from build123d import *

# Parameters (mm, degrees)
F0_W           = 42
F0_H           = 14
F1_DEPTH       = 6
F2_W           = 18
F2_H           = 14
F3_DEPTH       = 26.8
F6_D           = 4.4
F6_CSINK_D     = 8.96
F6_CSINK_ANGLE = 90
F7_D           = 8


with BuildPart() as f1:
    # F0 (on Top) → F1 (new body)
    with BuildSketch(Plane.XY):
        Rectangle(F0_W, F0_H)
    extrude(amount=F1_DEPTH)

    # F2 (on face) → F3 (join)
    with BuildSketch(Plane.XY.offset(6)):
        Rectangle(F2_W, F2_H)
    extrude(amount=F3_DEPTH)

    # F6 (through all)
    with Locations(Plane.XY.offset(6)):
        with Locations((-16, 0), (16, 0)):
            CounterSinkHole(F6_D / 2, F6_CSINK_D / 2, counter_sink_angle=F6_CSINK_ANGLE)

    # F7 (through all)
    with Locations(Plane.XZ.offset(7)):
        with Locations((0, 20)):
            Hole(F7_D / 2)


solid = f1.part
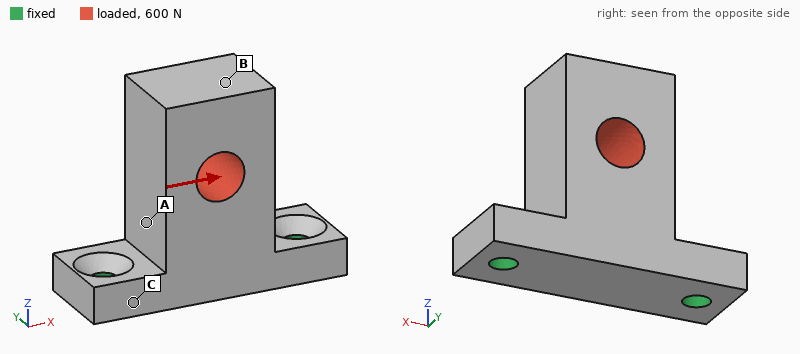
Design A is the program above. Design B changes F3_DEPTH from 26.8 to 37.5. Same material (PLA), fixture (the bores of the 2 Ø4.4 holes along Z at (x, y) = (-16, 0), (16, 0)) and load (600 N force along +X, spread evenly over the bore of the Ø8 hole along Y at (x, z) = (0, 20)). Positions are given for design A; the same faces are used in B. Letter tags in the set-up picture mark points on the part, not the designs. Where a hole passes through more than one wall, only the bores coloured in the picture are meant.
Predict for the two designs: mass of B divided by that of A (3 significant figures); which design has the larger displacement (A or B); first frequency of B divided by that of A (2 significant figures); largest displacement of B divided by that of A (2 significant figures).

1.29
B
0.62
1.3
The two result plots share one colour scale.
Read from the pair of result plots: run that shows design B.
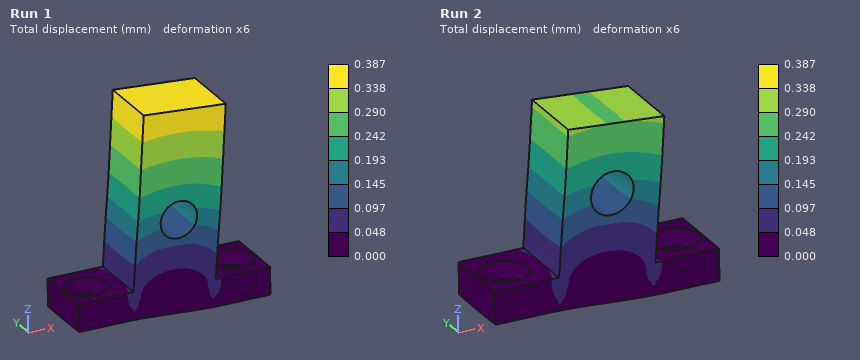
Run 1
